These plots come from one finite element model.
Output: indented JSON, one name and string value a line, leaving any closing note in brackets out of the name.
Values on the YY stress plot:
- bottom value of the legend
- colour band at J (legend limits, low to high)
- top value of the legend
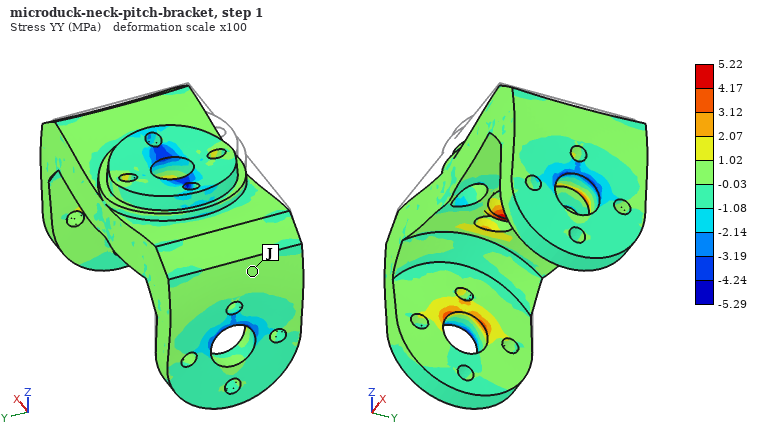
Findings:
{
  "bottom value of the legend": "-5.29 MPa",
  "colour band at J": "-0.03 to 1.02 MPa",
  "top value of the legend": "5.22 MPa"
}
